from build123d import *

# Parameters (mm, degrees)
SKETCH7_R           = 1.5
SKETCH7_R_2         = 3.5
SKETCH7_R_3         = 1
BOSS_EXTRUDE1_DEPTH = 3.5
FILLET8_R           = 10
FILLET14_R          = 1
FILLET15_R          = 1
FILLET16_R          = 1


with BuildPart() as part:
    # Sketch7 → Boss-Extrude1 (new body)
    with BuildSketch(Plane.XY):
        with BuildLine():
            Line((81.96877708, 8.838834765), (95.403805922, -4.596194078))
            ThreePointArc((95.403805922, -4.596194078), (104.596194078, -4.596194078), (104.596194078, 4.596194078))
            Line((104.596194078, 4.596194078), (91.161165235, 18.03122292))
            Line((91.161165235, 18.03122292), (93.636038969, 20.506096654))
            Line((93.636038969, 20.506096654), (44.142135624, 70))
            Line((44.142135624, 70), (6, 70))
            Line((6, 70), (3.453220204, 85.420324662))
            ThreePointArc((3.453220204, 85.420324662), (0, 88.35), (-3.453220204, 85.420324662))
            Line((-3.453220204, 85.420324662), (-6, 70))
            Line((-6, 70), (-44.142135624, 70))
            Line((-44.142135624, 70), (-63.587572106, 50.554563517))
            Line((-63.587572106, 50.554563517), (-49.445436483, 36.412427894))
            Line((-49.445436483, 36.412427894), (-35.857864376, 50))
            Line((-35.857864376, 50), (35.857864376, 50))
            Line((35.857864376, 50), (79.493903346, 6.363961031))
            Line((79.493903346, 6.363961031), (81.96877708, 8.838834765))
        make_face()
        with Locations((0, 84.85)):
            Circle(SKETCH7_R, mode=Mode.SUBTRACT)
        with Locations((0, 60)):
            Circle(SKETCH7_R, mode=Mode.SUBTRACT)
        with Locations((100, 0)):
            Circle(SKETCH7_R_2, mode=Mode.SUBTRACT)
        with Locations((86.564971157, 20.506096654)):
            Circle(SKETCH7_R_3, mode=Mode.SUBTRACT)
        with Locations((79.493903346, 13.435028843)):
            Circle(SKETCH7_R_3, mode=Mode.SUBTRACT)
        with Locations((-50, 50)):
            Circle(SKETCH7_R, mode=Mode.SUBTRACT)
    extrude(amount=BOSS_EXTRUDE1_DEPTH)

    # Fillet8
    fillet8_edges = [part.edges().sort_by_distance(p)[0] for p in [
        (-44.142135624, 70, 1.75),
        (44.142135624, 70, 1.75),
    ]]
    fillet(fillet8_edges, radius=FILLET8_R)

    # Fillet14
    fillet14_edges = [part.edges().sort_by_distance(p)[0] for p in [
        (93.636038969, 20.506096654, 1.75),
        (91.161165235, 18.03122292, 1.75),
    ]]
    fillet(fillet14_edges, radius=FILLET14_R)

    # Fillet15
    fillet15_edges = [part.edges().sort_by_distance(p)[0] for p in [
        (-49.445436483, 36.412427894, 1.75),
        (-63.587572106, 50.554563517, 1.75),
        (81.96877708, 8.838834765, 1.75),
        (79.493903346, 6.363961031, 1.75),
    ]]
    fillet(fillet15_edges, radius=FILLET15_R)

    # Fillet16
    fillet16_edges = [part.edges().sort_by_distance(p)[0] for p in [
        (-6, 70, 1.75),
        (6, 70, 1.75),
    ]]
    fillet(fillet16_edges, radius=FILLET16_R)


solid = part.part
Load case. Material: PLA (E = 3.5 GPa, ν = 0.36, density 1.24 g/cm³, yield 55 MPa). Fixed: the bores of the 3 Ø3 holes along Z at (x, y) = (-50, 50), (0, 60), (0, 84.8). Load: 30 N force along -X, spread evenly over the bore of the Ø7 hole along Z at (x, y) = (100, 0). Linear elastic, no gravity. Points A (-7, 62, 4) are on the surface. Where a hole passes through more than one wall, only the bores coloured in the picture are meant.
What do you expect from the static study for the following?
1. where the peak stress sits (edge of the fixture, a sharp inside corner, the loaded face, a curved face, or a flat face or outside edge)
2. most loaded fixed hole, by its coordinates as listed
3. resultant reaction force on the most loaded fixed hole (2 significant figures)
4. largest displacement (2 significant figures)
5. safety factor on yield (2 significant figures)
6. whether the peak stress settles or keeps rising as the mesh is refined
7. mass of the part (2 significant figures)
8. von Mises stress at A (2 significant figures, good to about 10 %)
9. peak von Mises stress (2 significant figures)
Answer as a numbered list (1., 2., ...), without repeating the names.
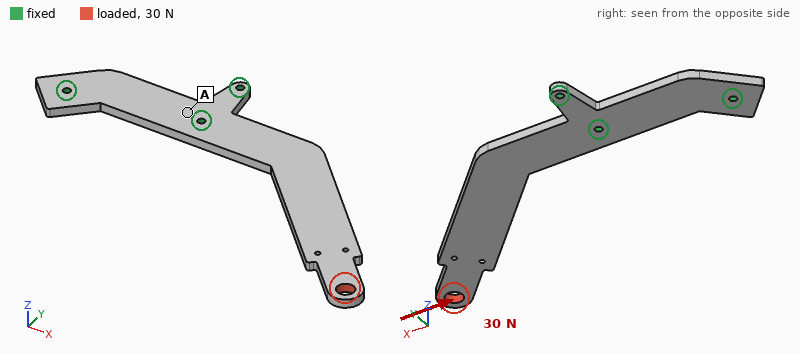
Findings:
1. a curved face
2. (0, 60)
3. 70 N
4. 1.8 mm
5. 2.5
6. settles
7. 16 g
8. 1.3 MPa
9. 22 MPa
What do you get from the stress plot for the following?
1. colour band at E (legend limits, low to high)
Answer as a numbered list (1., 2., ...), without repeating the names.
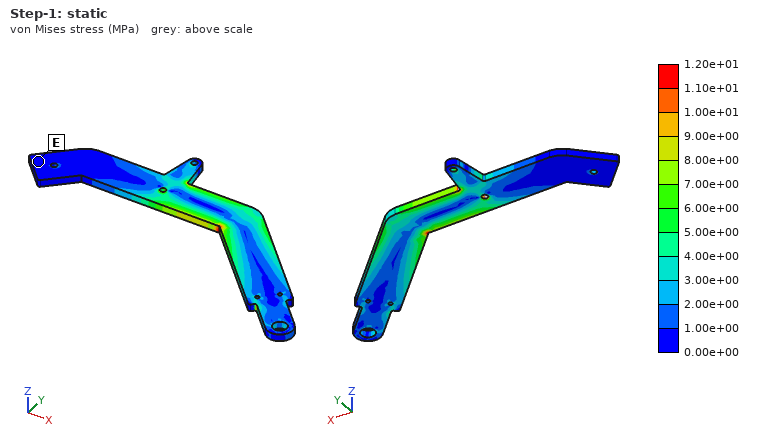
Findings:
1. 0.00e+00 to 1.00e+00 MPa
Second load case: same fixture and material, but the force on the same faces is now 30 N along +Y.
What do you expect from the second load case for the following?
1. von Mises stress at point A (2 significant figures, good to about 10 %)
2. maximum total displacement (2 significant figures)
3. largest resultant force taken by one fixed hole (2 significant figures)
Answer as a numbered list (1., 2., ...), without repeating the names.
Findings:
1. 2.0 MPa
2. 2.2 mm
3. 73 N
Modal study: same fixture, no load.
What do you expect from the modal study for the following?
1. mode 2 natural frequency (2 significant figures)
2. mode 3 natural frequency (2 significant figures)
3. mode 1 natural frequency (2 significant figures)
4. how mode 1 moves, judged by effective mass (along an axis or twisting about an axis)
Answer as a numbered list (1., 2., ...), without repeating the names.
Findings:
1. 350 Hz
2. 350 Hz
3. 72 Hz
4. along Z
